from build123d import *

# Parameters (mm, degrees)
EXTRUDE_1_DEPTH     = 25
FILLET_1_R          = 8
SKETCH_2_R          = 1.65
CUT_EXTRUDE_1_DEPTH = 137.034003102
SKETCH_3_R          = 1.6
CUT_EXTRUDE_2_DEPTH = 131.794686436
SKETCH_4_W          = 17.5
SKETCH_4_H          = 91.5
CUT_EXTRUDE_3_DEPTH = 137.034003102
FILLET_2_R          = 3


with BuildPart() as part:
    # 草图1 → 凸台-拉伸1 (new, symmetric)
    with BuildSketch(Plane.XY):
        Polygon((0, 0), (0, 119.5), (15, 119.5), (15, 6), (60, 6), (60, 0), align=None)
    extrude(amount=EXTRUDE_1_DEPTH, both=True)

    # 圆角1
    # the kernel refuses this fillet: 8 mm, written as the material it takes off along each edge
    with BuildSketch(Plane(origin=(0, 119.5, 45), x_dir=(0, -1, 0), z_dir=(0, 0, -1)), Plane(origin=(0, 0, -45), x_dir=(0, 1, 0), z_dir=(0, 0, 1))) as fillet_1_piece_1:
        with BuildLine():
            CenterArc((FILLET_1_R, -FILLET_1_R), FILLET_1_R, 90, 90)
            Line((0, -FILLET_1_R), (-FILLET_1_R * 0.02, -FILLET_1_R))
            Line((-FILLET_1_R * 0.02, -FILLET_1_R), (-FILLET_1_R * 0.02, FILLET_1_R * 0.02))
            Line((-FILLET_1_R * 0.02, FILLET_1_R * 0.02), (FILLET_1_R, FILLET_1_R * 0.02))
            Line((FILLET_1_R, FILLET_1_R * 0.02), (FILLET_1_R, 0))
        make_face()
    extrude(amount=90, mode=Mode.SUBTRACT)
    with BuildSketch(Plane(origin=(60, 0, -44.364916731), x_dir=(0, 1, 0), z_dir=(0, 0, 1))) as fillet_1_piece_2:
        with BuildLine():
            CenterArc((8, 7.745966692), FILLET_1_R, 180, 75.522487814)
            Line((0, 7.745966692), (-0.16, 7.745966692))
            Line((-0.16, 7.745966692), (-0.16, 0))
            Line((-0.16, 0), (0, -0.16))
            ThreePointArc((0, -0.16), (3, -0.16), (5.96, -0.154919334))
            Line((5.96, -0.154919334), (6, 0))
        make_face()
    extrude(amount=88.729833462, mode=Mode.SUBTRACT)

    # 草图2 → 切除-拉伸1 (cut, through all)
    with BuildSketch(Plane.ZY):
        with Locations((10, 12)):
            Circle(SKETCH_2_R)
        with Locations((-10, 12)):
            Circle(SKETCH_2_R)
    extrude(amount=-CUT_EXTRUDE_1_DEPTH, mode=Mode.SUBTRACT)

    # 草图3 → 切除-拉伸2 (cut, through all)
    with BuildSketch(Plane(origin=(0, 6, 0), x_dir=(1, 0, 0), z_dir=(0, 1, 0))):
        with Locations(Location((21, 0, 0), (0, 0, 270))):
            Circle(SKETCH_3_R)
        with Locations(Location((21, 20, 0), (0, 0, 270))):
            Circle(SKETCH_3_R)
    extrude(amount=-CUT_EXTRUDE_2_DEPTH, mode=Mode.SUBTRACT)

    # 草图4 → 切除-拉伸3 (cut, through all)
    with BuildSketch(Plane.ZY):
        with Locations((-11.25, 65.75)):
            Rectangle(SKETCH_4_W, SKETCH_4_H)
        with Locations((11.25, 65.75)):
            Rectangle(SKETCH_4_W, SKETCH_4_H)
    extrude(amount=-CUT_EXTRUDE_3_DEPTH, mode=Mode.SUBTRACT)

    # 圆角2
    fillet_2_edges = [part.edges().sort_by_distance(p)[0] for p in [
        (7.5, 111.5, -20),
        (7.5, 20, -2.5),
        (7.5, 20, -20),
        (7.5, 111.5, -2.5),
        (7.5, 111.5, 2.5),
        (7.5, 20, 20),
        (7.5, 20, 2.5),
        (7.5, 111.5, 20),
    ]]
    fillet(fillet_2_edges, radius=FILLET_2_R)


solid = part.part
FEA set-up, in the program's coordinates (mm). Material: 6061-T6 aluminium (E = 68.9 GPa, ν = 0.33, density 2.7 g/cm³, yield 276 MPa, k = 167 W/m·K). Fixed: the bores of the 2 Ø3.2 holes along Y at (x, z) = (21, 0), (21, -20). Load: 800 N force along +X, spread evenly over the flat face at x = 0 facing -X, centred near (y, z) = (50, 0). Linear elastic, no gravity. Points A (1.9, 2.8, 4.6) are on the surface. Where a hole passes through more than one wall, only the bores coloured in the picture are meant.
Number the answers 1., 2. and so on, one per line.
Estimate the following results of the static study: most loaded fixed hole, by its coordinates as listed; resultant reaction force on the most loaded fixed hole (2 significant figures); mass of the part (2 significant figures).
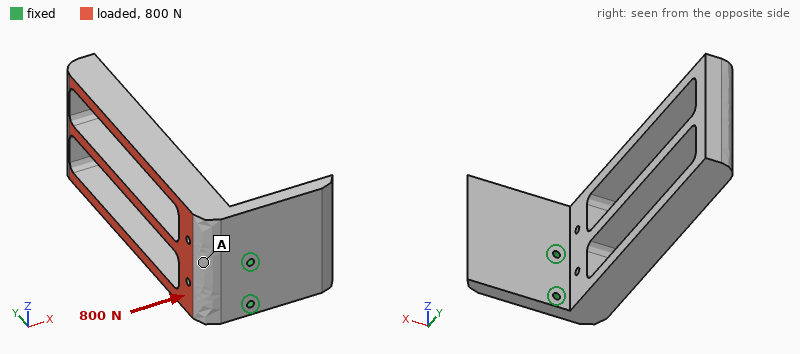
1. (21, 0)
2. 770 N
3. 140 g
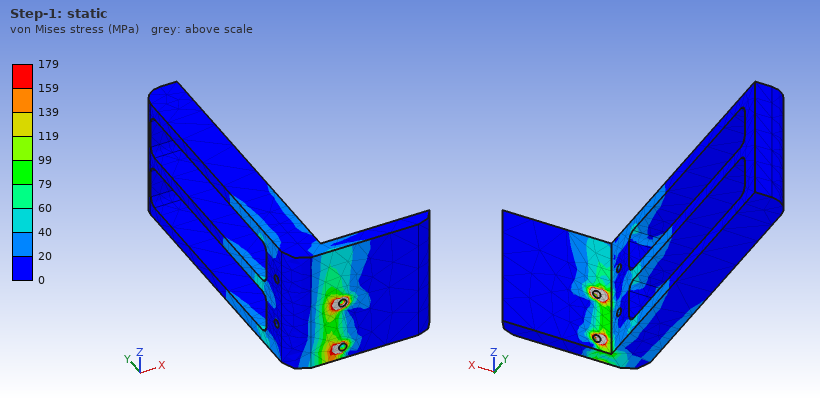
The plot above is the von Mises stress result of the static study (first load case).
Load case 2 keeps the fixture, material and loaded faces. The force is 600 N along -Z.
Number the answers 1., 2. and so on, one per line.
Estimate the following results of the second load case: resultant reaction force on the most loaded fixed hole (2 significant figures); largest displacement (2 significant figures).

1. 1.4 kN
2. 0.58 mm
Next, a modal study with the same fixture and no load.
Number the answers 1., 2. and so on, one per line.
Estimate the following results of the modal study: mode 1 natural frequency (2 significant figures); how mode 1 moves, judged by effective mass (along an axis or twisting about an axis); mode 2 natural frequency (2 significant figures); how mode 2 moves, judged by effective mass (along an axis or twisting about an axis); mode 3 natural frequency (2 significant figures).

1. 450 Hz
2. along X
3. 520 Hz
4. along Z
5. 1600 Hz
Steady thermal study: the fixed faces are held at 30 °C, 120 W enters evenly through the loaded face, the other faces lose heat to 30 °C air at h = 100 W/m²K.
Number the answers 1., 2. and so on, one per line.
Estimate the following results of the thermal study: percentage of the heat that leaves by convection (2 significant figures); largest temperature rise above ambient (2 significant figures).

1. 52 %
2. 54 K
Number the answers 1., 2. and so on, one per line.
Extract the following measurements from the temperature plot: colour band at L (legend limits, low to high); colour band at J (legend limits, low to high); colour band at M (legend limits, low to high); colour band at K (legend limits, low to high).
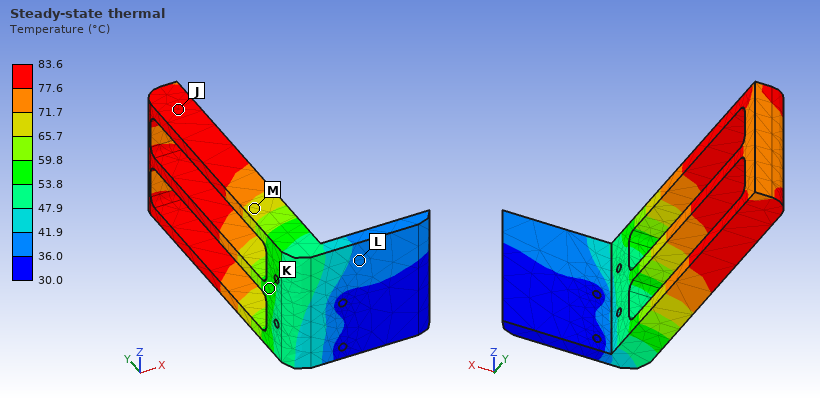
1. 36.0 to 41.9 °C
2. 77.6 to 83.6 °C
3. 65.7 to 71.7 °C
4. 53.8 to 59.8 °C
